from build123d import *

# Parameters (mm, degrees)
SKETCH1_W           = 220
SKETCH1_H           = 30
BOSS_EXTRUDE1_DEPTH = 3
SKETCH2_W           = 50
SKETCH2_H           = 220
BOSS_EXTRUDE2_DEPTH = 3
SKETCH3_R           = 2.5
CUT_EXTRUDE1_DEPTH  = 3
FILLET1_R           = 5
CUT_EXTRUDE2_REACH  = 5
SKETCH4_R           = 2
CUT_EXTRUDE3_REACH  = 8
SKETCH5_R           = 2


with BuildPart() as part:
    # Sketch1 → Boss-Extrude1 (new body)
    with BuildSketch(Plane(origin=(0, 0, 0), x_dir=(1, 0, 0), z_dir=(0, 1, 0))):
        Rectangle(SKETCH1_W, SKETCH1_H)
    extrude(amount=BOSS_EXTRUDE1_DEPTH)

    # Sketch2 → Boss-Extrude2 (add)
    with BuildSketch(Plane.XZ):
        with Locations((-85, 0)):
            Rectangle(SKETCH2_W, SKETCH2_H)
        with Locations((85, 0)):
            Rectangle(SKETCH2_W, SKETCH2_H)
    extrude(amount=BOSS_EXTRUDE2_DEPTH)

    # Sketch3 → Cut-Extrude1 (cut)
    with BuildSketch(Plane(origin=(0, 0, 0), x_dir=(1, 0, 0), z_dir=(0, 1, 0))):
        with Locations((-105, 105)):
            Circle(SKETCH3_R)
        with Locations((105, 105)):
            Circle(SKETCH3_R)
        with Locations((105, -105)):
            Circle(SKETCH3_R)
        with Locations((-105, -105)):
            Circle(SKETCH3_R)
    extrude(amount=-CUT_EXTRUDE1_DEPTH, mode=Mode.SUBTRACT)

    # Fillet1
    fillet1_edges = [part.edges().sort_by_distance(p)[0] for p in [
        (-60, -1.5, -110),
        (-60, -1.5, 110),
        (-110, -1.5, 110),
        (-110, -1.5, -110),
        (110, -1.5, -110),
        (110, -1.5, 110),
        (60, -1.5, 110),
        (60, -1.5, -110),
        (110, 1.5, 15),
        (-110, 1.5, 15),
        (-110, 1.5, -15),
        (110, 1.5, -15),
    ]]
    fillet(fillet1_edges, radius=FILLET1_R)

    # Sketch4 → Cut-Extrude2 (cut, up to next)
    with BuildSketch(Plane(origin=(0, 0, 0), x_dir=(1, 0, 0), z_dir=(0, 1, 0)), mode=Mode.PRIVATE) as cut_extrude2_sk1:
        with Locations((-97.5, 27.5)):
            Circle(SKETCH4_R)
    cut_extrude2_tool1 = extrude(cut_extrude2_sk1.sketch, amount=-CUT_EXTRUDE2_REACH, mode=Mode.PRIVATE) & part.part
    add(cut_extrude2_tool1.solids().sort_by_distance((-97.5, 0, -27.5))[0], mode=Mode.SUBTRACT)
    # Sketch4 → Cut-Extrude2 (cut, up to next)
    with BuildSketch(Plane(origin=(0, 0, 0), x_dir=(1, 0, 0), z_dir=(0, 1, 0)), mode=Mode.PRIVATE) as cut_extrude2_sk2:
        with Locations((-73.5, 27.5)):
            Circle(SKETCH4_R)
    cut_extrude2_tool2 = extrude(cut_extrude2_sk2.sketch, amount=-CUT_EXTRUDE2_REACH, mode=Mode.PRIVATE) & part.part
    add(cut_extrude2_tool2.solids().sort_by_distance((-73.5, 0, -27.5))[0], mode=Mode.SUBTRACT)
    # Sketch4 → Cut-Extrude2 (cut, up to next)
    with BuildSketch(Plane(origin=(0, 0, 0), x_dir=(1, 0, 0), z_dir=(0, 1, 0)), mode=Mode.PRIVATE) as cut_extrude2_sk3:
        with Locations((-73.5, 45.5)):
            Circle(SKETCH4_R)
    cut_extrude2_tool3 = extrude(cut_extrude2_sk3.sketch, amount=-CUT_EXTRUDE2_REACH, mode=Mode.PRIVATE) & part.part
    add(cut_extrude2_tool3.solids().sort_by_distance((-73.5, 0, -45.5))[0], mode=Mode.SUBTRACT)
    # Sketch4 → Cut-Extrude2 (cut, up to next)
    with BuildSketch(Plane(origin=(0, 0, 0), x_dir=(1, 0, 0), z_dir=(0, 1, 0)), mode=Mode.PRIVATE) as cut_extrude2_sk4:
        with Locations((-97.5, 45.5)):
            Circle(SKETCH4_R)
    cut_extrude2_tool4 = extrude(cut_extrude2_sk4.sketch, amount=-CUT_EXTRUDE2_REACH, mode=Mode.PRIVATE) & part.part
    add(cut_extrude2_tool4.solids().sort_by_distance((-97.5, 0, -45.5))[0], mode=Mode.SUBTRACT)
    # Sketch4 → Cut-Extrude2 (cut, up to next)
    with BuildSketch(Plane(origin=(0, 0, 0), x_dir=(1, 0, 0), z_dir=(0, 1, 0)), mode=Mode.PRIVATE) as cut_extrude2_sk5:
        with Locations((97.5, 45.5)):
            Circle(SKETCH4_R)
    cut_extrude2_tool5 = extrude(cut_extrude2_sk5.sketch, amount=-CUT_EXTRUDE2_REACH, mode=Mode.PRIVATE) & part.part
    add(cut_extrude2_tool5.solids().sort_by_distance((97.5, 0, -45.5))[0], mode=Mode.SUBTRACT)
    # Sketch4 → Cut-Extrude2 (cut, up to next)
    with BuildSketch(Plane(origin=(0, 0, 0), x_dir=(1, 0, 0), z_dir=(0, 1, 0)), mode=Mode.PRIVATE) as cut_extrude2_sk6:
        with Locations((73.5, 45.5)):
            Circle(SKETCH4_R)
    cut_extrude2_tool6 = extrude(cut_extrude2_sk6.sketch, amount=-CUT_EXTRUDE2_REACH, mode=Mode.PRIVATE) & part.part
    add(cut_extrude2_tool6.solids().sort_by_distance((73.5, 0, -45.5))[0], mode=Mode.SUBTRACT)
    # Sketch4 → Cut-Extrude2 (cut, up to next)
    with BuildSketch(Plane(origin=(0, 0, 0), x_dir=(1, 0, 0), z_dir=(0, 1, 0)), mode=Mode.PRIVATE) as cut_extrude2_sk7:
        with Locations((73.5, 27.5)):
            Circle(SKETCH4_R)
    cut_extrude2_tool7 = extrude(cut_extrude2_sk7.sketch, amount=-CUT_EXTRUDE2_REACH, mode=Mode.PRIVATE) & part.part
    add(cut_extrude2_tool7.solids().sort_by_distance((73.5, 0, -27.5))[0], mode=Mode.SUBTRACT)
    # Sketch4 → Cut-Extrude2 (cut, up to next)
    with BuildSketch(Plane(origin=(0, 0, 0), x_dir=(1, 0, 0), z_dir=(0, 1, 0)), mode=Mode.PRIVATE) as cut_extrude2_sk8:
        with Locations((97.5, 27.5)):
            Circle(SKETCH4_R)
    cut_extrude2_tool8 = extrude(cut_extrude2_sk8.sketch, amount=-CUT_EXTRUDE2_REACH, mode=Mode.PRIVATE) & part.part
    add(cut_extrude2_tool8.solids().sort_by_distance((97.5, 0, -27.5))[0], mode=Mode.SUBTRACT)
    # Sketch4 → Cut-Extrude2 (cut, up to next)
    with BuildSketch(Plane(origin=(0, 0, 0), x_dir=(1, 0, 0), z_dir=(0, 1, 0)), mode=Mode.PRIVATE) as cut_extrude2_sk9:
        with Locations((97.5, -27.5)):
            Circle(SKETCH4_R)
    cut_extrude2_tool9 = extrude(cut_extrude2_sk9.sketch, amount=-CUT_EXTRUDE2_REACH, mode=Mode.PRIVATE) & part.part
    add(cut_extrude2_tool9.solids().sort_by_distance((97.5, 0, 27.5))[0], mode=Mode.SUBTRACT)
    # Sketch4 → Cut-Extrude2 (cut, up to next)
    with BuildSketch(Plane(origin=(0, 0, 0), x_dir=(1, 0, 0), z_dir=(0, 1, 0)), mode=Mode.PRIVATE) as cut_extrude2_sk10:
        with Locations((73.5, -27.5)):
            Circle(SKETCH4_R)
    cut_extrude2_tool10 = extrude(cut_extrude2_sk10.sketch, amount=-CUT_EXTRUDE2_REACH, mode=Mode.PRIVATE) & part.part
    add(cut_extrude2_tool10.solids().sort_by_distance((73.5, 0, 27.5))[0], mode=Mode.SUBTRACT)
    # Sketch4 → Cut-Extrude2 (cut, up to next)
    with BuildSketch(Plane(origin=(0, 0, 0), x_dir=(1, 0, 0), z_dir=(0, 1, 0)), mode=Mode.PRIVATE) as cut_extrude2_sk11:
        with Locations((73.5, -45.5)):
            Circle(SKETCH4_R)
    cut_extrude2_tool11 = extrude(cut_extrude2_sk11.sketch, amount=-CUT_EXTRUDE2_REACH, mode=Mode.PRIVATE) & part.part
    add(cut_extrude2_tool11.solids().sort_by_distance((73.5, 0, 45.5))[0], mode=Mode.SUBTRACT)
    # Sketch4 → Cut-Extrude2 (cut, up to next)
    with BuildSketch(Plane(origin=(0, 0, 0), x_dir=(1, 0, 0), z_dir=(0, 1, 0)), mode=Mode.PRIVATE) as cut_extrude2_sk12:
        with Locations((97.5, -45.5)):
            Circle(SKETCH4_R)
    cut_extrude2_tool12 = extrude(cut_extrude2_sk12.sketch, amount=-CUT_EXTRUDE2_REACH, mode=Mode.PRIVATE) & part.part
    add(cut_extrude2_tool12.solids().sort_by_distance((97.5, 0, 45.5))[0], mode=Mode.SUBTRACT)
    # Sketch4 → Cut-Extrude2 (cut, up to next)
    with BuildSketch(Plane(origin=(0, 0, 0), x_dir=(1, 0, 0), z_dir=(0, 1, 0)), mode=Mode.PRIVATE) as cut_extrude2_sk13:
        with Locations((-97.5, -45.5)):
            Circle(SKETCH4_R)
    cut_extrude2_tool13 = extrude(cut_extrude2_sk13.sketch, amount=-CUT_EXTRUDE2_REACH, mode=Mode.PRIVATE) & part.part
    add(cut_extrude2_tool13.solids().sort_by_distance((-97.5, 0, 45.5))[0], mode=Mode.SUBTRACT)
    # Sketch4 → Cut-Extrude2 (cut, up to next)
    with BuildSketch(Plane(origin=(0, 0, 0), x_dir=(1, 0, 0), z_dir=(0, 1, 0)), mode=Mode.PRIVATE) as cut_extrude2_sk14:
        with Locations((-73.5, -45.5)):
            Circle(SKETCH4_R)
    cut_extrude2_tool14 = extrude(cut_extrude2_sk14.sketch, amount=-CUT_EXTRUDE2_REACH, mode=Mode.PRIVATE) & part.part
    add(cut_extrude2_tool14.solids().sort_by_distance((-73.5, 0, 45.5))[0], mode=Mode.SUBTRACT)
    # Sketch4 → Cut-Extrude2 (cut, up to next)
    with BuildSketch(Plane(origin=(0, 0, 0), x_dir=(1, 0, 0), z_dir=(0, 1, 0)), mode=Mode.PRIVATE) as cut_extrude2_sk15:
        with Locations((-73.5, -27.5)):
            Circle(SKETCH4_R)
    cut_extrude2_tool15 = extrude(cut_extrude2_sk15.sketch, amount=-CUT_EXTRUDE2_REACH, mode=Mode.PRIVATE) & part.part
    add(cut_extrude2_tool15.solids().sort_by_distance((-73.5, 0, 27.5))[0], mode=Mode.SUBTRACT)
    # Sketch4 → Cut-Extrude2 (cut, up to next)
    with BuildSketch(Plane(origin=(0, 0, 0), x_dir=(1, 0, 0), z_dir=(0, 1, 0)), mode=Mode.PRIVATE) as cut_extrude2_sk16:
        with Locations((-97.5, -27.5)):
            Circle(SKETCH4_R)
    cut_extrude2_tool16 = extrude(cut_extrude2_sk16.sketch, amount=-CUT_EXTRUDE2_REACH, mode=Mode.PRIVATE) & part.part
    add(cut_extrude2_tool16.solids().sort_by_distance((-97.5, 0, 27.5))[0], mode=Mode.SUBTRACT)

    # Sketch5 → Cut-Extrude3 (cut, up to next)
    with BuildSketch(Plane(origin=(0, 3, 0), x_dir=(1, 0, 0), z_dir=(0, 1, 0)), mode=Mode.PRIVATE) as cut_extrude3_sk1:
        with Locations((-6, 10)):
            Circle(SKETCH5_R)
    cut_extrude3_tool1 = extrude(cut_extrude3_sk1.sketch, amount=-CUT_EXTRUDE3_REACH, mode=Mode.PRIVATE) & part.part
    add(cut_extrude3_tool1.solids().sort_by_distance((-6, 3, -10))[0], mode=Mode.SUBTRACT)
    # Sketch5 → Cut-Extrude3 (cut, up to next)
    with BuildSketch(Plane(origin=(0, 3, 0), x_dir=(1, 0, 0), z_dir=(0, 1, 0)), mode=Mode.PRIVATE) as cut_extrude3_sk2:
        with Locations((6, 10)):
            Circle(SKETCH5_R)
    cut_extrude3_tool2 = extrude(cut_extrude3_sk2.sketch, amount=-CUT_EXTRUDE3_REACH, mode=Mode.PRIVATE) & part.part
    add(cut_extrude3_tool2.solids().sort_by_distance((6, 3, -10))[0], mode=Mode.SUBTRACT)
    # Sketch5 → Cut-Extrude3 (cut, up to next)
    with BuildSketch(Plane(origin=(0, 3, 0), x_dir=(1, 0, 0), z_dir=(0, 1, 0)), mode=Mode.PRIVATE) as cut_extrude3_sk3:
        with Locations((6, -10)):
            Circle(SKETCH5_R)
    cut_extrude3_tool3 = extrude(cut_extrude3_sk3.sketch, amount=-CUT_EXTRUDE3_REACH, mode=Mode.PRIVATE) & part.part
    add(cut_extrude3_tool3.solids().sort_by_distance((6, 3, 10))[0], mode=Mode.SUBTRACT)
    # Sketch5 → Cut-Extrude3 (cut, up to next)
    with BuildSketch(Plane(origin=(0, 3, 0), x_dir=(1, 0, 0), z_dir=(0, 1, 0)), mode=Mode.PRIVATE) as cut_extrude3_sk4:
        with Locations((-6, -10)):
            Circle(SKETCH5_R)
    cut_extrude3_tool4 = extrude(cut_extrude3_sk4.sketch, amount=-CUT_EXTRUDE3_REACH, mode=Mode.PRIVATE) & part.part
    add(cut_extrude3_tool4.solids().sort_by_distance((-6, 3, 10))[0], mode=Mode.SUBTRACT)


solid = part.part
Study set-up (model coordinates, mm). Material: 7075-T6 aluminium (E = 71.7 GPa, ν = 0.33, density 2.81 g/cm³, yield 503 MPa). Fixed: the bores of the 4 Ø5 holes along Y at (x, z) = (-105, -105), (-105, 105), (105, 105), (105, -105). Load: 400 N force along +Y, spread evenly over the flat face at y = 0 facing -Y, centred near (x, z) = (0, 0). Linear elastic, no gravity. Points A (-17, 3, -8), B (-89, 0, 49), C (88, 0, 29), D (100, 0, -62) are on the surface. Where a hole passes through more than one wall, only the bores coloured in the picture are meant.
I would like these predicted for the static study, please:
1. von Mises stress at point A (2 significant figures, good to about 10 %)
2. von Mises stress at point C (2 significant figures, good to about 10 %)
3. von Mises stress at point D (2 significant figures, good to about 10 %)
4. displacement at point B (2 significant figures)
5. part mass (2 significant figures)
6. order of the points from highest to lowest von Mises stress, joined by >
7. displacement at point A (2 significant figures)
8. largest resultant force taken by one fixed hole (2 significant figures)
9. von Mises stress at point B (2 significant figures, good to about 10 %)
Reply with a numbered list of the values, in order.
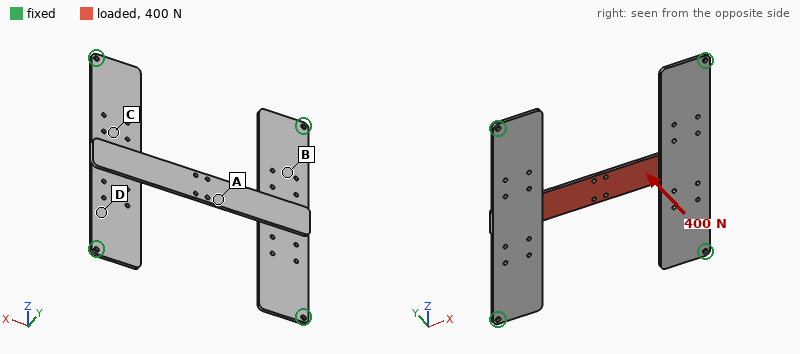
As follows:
1. 87 MPa
2. 52 MPa
3. 16 MPa
4. 0.94 mm
5. 240 g
6. A > C > B > D
7. 3.0 mm
8. 1.2 kN
9. 29 MPa
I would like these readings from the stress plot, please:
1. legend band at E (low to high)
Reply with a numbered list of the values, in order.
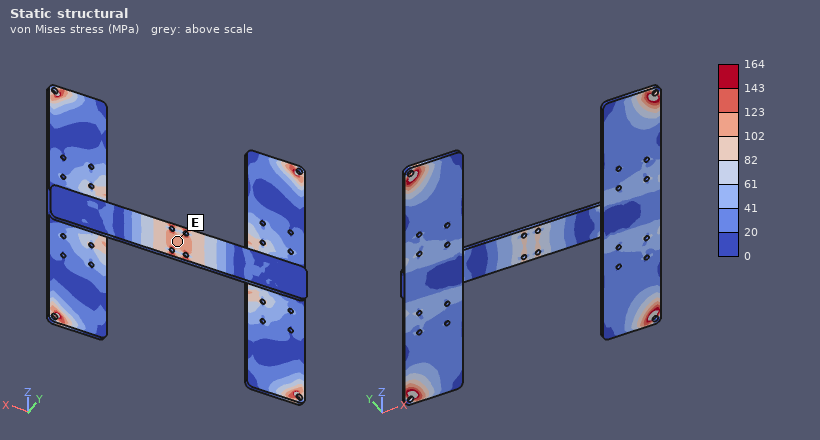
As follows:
1. 102 to 123 MPa
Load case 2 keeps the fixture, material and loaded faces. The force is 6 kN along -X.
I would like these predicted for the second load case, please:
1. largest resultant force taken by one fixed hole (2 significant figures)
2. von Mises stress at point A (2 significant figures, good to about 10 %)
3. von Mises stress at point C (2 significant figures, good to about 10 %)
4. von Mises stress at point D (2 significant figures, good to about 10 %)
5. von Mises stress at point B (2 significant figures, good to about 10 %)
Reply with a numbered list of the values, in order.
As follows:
1. 2.7 kN
2. 26 MPa
3. 45 MPa
4. 39 MPa
5. 46 MPa
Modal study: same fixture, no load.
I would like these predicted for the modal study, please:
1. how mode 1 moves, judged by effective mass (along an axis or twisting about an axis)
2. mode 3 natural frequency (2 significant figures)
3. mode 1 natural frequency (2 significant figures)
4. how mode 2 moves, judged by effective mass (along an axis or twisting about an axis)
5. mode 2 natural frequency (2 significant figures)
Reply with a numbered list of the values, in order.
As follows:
1. along Y
2. 560 Hz
3. 230 Hz
4. twisting about Z
5. 300 Hz
